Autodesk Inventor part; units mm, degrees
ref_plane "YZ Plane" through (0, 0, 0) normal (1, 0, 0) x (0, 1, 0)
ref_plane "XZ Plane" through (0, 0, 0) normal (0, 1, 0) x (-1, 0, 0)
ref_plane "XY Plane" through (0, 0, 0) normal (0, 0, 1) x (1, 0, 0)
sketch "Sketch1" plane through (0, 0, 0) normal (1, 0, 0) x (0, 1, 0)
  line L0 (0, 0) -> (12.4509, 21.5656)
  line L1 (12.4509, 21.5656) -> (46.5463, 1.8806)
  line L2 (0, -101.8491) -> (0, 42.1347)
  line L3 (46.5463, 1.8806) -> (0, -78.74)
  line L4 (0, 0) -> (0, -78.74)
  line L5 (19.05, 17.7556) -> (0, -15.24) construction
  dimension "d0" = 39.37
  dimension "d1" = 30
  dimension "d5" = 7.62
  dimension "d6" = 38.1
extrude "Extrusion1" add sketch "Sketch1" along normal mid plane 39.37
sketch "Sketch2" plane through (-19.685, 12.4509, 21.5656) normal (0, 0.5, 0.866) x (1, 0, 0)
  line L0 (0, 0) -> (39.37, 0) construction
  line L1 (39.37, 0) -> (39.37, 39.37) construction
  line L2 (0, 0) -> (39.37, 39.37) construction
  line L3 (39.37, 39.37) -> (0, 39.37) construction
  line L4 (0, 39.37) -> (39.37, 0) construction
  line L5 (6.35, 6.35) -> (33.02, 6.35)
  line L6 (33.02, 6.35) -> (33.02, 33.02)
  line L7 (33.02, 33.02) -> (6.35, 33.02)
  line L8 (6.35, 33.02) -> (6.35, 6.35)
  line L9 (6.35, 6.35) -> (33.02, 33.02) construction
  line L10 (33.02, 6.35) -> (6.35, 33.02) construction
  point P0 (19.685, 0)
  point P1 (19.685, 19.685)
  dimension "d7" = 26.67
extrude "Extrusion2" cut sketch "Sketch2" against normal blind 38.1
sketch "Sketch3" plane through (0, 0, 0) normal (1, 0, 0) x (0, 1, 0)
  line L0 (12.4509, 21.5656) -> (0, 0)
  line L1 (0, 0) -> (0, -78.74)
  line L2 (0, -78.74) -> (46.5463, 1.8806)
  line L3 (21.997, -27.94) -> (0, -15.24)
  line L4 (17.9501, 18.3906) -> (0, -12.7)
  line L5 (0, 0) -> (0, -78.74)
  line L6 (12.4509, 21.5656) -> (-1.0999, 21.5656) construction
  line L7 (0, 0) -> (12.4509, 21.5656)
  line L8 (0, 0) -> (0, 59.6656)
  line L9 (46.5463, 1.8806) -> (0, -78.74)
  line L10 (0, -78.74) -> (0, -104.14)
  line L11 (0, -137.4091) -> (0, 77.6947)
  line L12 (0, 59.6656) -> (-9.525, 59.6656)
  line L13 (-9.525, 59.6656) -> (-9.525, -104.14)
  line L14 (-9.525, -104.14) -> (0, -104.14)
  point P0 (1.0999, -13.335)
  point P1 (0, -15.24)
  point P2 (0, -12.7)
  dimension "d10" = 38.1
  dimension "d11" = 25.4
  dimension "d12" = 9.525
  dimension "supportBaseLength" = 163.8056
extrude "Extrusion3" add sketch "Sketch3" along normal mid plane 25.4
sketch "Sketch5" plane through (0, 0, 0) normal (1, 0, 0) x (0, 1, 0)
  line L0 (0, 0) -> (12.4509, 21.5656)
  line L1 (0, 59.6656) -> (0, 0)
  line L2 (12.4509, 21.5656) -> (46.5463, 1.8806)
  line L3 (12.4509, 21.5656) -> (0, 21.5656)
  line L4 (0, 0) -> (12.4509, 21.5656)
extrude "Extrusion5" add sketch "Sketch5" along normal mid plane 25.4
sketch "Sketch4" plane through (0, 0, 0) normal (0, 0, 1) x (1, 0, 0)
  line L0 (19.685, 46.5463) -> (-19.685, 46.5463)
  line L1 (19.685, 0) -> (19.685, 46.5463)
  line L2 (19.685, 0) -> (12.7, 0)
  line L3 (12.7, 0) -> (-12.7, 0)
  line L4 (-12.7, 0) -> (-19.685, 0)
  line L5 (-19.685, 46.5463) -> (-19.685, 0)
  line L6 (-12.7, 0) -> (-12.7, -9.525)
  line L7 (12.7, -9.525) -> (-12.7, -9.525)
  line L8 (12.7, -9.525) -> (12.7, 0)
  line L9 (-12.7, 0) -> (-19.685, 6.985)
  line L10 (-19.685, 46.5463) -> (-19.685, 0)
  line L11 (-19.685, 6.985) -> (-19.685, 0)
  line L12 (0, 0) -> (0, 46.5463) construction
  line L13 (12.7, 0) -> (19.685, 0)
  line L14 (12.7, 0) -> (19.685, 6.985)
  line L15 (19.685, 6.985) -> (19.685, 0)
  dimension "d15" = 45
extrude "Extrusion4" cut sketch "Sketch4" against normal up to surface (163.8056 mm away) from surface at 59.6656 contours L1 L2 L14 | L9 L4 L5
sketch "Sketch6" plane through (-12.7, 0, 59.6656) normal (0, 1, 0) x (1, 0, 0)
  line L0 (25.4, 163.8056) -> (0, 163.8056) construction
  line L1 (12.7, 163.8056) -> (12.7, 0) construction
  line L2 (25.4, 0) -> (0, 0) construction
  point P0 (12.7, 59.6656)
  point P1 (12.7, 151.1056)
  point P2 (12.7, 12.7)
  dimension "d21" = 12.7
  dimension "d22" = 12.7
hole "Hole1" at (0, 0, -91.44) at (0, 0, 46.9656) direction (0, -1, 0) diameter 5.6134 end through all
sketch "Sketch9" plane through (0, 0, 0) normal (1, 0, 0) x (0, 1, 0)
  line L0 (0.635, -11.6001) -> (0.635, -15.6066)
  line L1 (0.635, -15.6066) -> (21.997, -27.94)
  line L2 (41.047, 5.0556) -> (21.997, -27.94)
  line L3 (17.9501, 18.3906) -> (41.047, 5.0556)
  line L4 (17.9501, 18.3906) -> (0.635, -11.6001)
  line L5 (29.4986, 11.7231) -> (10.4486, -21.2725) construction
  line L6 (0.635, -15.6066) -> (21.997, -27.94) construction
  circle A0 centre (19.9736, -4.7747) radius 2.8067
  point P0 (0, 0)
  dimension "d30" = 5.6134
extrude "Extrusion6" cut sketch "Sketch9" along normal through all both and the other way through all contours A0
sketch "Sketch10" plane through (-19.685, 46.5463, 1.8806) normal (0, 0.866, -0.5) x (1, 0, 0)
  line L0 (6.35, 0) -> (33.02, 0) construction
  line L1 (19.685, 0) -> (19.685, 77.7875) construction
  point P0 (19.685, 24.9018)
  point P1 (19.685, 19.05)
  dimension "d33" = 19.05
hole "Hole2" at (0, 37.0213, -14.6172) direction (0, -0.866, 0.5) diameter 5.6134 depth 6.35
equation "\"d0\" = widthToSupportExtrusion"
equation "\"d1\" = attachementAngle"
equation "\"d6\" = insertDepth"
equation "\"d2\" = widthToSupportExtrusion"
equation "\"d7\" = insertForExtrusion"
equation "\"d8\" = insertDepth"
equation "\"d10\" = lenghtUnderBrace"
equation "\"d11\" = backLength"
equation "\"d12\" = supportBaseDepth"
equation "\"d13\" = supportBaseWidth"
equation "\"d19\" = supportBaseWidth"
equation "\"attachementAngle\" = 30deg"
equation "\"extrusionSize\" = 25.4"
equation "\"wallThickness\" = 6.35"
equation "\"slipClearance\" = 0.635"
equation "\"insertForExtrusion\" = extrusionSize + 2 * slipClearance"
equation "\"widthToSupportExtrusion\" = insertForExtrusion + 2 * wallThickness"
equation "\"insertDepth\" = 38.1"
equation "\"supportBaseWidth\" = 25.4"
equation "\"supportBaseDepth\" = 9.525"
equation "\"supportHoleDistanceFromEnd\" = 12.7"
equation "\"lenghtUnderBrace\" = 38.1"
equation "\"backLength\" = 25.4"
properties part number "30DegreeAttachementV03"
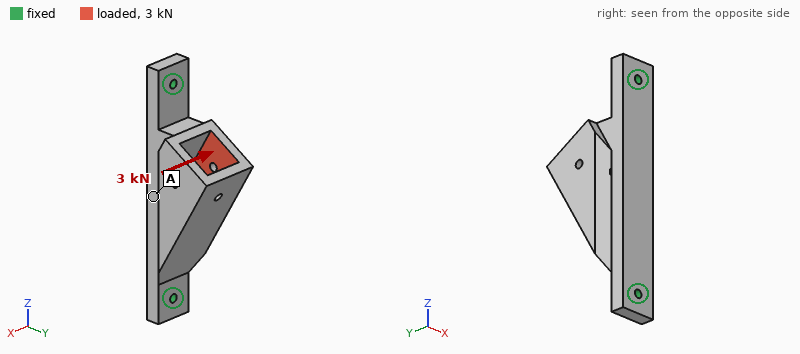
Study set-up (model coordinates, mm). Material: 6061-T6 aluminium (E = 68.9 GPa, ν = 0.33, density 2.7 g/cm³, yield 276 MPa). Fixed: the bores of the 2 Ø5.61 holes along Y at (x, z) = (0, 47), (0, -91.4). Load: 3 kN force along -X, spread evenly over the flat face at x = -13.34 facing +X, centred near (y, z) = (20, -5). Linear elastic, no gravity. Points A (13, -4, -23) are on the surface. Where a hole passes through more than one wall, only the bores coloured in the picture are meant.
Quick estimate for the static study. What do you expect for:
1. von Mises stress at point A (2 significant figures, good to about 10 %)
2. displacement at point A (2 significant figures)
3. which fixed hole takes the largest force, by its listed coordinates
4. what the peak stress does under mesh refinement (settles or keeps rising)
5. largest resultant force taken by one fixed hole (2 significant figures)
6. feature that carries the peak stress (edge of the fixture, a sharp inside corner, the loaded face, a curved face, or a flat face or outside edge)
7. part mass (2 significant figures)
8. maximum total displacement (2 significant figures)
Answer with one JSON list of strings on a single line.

["13 MPa", "0.085 mm", "(0, 47)", "keeps rising", "1.9 kN", "edge of the fixture", "280 g", "0.38 mm"]
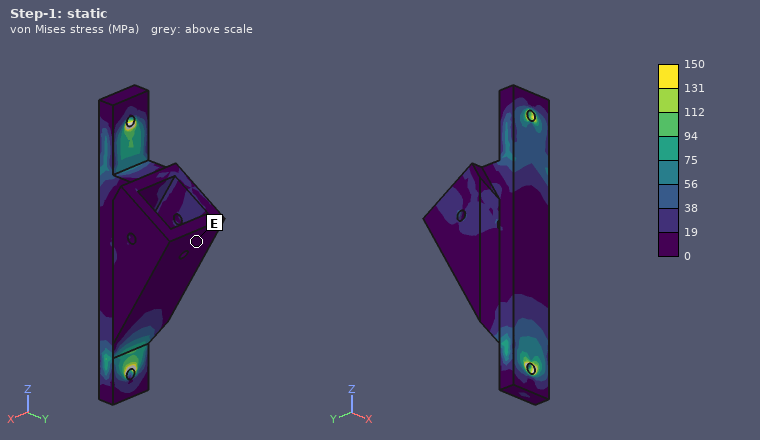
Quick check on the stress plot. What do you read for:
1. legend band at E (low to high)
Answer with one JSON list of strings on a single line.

["0 to 19 MPa"]
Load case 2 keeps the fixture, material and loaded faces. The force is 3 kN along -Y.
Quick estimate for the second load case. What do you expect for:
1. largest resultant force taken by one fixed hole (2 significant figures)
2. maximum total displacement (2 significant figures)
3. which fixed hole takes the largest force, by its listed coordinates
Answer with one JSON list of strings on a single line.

["2.4 kN", "0.20 mm", "(0, 47)"]
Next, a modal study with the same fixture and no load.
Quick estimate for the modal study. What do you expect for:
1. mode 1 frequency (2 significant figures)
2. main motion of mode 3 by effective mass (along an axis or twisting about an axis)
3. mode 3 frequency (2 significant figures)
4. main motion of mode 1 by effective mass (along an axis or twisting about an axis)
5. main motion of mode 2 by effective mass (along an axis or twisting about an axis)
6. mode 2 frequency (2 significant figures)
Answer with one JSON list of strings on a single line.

["1500 Hz", "along X", "4500 Hz", "along X", "along Y", "2900 Hz"]
